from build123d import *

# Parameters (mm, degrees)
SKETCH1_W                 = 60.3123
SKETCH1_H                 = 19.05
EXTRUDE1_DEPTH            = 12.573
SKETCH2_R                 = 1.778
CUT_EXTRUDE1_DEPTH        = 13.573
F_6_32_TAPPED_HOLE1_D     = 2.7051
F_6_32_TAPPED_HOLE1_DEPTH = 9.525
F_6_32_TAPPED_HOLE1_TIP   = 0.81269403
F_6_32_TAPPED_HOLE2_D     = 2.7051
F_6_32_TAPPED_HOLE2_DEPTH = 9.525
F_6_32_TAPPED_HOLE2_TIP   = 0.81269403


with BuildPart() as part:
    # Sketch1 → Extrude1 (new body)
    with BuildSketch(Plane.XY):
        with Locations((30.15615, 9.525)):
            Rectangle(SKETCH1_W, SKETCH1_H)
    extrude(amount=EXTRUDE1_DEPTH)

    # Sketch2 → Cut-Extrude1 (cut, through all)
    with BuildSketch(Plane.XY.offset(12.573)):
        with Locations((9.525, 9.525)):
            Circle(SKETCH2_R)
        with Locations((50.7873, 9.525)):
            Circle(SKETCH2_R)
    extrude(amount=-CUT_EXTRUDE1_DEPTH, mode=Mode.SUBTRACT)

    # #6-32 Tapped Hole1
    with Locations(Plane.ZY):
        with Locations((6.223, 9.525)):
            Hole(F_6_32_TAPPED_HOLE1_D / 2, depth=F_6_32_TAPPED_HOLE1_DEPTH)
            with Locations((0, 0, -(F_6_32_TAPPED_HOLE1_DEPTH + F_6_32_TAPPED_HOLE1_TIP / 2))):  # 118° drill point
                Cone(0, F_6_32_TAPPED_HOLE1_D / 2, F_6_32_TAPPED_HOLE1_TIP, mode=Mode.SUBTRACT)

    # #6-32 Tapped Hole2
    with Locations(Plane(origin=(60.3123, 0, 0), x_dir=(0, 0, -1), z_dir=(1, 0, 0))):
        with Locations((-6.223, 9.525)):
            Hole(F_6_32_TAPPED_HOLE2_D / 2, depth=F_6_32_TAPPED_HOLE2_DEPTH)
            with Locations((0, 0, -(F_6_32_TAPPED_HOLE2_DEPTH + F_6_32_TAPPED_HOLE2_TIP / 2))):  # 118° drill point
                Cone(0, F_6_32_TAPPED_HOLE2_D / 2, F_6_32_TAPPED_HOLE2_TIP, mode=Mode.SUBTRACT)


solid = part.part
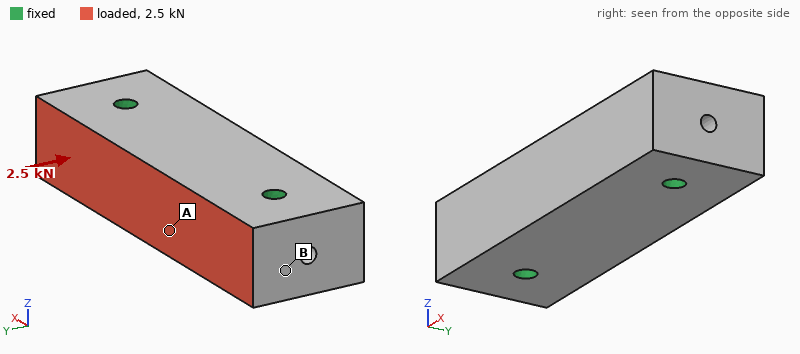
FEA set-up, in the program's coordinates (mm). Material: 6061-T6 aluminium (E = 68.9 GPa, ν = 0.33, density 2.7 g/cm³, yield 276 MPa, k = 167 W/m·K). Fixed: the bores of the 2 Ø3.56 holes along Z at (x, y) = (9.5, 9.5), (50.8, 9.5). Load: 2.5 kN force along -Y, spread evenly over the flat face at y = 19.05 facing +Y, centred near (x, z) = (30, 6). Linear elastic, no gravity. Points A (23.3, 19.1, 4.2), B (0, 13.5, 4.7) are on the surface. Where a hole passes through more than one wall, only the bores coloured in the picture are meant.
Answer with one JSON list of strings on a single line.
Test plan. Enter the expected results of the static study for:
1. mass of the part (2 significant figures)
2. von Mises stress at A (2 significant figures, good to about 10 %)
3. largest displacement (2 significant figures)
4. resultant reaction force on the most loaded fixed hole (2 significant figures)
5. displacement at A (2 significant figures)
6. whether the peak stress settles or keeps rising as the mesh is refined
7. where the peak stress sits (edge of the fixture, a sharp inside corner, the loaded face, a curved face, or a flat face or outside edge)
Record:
["38 g", "6.0 MPa", "3.4 µm", "1.3 kN", "3.0 µm", "keeps rising", "edge of the fixture"]
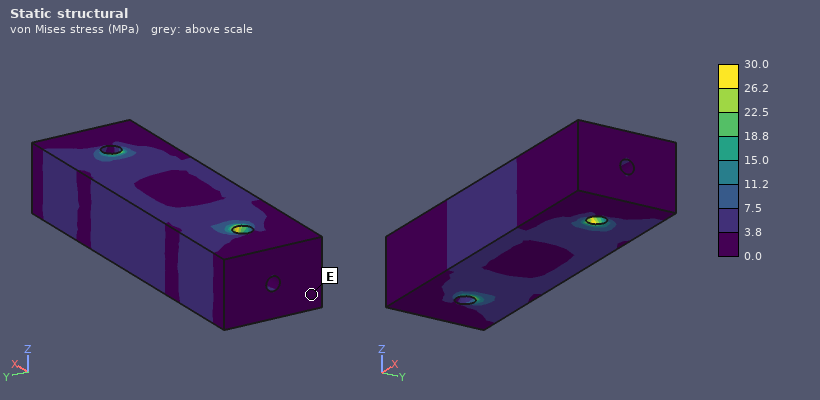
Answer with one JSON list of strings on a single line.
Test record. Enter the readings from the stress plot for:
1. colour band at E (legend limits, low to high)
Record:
["0.0 to 3.8 MPa"]
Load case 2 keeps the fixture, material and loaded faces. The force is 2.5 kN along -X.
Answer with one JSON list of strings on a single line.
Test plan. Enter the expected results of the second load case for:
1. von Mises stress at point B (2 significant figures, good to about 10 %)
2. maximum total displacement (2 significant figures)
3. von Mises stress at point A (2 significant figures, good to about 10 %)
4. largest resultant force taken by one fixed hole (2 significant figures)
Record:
["5.9 MPa", "3.8 µm", "5.7 MPa", "1.4 kN"]
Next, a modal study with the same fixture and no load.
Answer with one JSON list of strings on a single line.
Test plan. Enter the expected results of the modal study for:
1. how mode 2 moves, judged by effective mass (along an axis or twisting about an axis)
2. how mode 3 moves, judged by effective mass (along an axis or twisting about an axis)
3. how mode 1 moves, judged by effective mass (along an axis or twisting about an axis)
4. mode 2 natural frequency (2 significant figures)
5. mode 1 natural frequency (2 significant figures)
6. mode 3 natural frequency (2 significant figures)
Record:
["along Z", "twisting about X", "along Y", "23 kHz", "22 kHz", "28 kHz"]
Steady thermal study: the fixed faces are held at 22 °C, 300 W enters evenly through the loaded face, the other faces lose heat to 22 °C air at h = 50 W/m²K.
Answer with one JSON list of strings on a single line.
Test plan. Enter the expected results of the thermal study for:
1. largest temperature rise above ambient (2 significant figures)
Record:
["49 K"]
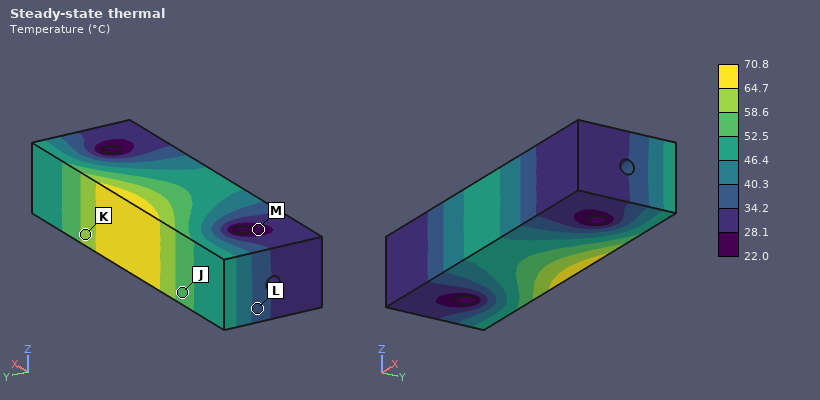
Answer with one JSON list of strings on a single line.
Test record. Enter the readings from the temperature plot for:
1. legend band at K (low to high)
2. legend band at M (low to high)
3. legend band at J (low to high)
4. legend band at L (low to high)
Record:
["58.6 to 64.7 °C", "22.0 to 28.1 °C", "52.5 to 58.6 °C", "34.2 to 40.3 °C"]
